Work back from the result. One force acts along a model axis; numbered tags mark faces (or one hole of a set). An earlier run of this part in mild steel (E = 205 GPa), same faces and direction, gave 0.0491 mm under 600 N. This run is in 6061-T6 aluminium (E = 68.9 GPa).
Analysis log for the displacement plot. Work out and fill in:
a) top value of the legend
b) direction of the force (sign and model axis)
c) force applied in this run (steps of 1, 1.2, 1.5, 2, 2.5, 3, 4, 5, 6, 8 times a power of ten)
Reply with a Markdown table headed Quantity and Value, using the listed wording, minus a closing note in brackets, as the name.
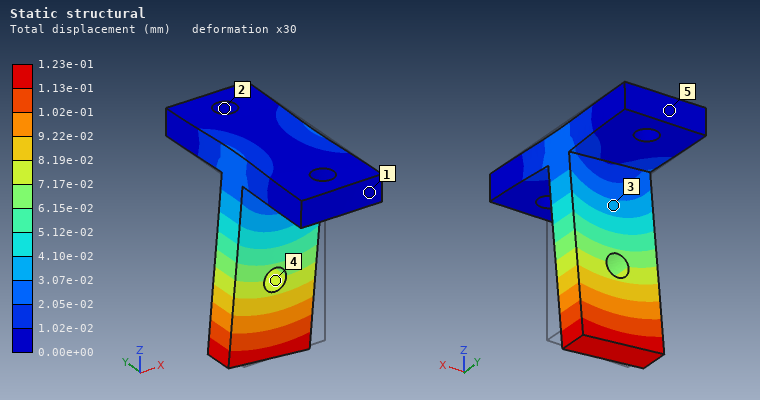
| Quantity | Value |
|---|---|
| top value of the legend | 1.23e-01 mm |
| direction of the force | -X |
| force applied in this run | 500 N |
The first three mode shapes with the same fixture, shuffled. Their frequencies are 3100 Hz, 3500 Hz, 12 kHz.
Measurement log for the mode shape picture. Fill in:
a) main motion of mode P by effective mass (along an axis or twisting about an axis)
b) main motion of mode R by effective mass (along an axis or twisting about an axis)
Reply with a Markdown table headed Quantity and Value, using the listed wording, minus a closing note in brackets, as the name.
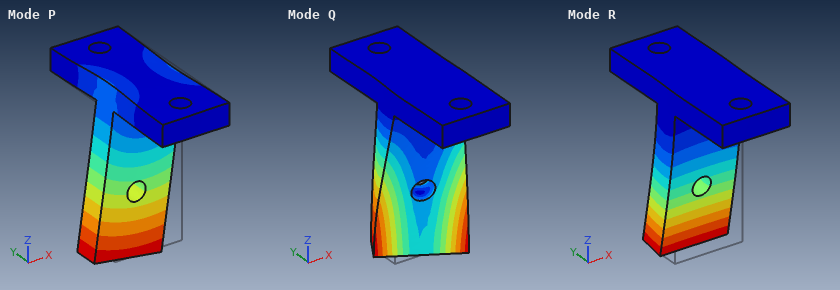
| Quantity | Value |
|---|---|
| main motion of mode P by effective mass | along X |
| main motion of mode R by effective mass | along Y |
